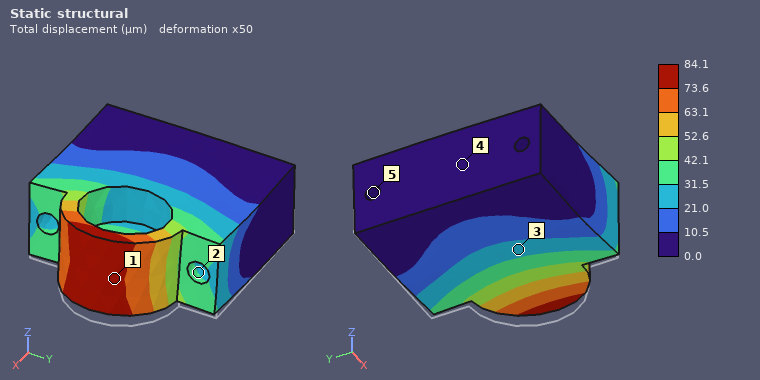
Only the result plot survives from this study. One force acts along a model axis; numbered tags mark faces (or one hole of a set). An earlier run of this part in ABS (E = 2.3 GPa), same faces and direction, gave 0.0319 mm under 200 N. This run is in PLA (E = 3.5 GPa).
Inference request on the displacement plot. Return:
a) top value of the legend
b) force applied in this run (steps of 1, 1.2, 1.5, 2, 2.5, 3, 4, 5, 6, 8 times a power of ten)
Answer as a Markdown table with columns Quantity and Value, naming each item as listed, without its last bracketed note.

| Quantity | Value |
|---|---|
| top value of the legend | 84.1 µm |
| force applied in this run | 800 N |
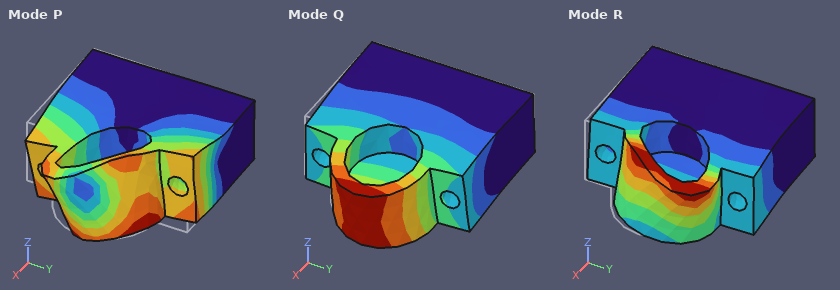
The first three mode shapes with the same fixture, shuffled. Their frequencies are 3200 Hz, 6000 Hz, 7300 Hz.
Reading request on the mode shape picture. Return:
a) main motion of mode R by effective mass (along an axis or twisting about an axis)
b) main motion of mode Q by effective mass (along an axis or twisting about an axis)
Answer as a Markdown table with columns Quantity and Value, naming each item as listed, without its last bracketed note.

| Quantity | Value |
|---|---|
| main motion of mode R by effective mass | along Y |
| main motion of mode Q by effective mass | along Z |
